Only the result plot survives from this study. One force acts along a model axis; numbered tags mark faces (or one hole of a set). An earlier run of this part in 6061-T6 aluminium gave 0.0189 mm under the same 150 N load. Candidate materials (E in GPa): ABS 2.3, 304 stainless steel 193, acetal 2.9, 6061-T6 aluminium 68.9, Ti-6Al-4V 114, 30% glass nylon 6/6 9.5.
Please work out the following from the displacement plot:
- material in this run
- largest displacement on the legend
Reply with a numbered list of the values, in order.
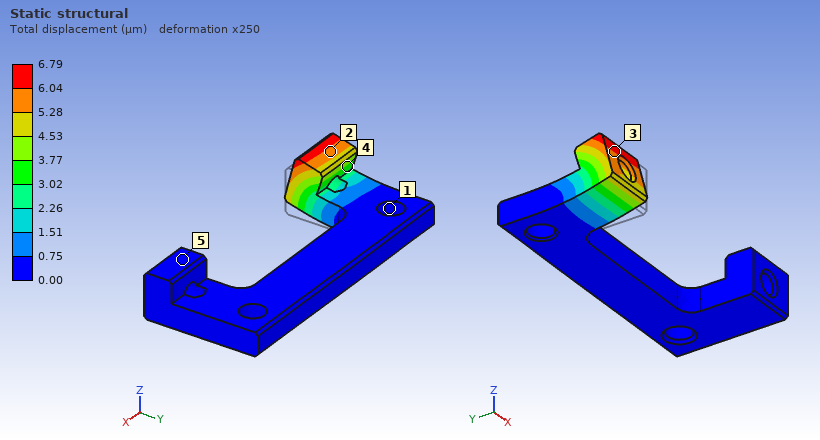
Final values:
1. 304 stainless steel
2. 6.79 µm
